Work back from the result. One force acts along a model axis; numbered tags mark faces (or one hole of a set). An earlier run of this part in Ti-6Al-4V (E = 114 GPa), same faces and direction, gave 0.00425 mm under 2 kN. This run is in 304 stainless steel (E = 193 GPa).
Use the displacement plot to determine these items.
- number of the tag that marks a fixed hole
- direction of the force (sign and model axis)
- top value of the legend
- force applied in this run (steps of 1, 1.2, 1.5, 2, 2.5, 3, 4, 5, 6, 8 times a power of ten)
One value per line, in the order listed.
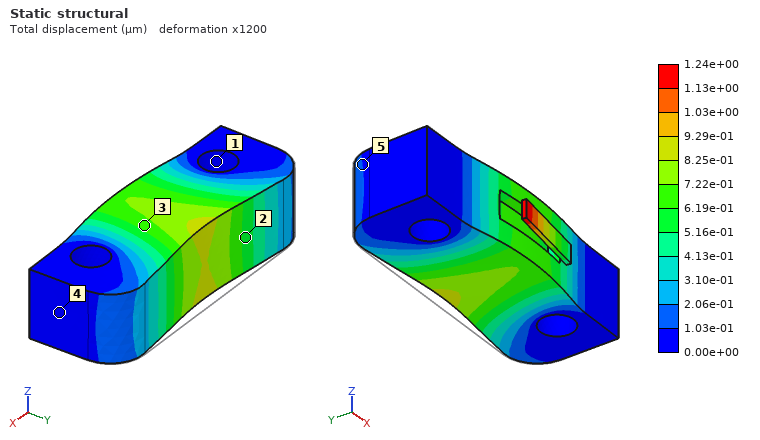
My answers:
1
-Y
1.24e+00 µm
1 kN
